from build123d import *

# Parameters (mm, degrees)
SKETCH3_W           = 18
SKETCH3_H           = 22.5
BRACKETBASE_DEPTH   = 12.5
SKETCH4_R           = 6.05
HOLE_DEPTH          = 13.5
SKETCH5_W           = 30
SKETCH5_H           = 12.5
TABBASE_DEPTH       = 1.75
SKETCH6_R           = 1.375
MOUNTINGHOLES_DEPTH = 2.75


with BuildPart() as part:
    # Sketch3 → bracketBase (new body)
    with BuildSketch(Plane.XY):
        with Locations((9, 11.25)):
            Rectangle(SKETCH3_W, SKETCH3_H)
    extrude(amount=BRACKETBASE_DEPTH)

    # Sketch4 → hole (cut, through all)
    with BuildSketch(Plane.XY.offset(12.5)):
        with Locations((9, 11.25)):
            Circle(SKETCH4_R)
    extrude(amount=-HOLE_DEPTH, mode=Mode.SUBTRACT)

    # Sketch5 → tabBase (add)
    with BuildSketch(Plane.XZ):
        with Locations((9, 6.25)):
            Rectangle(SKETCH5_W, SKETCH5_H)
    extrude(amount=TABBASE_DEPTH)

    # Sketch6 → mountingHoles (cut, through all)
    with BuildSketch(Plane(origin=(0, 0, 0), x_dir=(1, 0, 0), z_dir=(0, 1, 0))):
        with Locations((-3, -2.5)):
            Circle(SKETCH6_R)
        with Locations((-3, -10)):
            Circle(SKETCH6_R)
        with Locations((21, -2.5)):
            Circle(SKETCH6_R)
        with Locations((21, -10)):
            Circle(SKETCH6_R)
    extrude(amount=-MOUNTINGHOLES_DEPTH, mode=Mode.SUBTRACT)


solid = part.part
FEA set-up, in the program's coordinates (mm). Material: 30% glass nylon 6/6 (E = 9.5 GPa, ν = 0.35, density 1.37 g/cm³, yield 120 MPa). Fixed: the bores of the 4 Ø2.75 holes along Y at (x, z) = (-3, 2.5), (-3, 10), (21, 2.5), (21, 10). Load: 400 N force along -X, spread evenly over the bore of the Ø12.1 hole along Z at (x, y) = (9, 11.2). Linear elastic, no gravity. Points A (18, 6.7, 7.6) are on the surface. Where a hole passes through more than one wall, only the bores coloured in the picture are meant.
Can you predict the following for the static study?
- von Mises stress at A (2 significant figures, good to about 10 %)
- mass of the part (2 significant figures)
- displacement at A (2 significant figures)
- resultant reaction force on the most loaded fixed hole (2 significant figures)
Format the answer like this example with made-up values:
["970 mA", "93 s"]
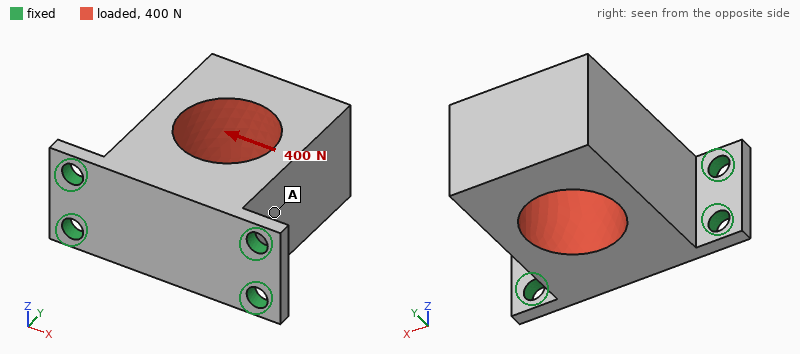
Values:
["12 MPa", "5.8 g", "0.037 mm", "160 N"]
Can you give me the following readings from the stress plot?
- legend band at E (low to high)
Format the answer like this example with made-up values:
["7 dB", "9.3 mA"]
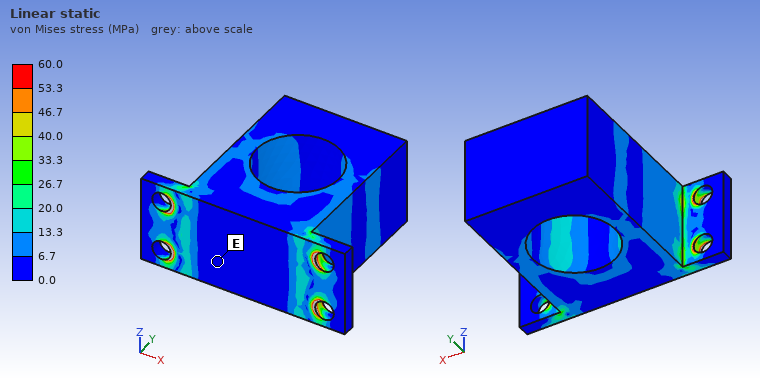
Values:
["0.0 to 6.7 MPa"]
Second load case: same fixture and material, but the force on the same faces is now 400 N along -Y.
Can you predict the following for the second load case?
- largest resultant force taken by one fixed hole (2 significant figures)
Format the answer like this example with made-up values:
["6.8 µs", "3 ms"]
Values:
["110 N"]
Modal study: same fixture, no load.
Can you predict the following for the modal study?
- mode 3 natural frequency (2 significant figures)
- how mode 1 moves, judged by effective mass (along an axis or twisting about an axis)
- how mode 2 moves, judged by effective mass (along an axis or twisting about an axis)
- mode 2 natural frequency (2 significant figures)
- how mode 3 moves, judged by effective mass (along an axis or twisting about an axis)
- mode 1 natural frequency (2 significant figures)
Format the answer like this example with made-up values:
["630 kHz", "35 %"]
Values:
["9100 Hz", "along Z", "along X", "5000 Hz", "along Y", "2600 Hz"]
